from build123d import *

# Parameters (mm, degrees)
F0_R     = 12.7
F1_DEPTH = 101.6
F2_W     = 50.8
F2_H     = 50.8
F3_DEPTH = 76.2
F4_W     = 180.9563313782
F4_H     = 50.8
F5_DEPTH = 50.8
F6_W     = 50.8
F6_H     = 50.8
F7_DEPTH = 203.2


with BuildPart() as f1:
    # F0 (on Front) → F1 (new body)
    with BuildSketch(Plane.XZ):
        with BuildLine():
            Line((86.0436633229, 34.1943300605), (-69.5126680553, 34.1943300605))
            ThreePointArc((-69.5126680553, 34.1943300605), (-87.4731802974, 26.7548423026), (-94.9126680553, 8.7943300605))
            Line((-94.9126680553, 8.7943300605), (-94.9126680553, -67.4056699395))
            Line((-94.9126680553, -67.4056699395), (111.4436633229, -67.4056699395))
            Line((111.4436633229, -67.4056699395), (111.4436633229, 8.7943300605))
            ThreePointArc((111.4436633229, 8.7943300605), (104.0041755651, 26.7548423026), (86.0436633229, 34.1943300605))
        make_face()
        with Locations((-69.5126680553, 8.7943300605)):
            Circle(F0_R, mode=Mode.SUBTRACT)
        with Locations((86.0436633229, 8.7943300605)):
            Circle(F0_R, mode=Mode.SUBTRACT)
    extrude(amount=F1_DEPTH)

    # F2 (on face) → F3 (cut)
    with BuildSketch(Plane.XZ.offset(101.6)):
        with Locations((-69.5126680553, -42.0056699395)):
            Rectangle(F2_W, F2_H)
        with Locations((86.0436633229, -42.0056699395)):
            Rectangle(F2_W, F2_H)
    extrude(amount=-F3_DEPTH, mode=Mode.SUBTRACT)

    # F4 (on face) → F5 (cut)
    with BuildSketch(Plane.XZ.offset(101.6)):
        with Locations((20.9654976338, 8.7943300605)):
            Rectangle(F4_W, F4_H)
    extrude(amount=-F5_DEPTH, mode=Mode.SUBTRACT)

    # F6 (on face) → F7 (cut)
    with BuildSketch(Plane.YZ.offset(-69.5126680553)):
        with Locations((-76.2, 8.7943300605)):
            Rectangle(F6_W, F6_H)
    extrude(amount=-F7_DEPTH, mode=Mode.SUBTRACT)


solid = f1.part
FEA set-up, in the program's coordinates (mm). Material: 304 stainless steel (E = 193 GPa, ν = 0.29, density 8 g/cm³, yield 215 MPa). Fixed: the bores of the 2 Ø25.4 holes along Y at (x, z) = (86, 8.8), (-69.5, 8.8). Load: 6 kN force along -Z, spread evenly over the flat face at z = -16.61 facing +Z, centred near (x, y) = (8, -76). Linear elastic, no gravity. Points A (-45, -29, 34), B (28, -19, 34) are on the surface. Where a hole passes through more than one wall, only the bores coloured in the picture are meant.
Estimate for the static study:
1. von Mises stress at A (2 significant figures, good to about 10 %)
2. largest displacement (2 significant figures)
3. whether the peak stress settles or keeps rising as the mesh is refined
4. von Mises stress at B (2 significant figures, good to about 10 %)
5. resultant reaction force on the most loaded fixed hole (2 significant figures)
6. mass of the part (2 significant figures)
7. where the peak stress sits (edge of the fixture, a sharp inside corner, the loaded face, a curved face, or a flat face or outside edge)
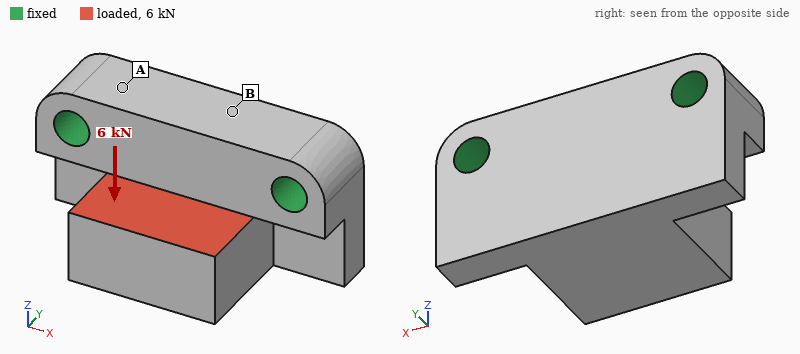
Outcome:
5.1 MPa
10 µm
keeps rising
2.3 MPa
3.2 kN
9.1 kg
a sharp inside corner
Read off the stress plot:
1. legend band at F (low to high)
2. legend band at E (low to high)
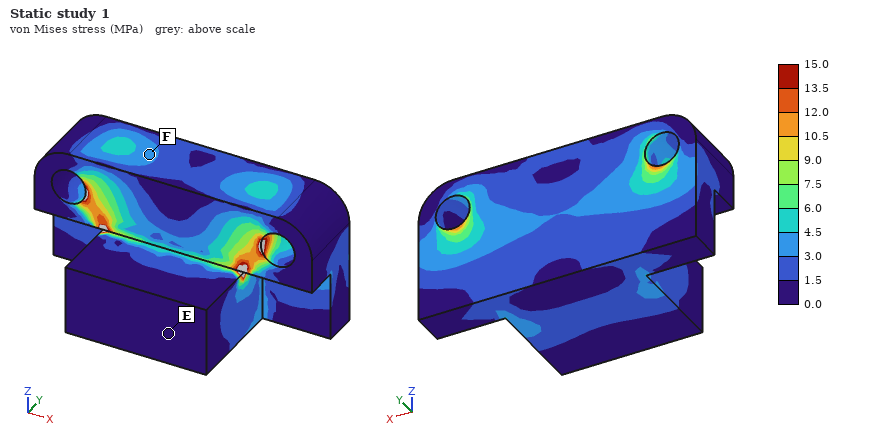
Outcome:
3.0 to 4.5 MPa
0.0 to 1.5 MPa
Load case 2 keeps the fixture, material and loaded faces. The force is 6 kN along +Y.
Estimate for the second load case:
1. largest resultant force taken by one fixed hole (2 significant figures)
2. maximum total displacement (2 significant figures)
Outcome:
3.0 kN
2.4 µm
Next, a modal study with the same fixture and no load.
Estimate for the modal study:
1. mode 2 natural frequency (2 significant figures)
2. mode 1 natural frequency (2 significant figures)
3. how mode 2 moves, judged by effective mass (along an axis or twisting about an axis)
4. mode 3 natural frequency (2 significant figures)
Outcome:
4600 Hz
2300 Hz
along X
5200 Hz
